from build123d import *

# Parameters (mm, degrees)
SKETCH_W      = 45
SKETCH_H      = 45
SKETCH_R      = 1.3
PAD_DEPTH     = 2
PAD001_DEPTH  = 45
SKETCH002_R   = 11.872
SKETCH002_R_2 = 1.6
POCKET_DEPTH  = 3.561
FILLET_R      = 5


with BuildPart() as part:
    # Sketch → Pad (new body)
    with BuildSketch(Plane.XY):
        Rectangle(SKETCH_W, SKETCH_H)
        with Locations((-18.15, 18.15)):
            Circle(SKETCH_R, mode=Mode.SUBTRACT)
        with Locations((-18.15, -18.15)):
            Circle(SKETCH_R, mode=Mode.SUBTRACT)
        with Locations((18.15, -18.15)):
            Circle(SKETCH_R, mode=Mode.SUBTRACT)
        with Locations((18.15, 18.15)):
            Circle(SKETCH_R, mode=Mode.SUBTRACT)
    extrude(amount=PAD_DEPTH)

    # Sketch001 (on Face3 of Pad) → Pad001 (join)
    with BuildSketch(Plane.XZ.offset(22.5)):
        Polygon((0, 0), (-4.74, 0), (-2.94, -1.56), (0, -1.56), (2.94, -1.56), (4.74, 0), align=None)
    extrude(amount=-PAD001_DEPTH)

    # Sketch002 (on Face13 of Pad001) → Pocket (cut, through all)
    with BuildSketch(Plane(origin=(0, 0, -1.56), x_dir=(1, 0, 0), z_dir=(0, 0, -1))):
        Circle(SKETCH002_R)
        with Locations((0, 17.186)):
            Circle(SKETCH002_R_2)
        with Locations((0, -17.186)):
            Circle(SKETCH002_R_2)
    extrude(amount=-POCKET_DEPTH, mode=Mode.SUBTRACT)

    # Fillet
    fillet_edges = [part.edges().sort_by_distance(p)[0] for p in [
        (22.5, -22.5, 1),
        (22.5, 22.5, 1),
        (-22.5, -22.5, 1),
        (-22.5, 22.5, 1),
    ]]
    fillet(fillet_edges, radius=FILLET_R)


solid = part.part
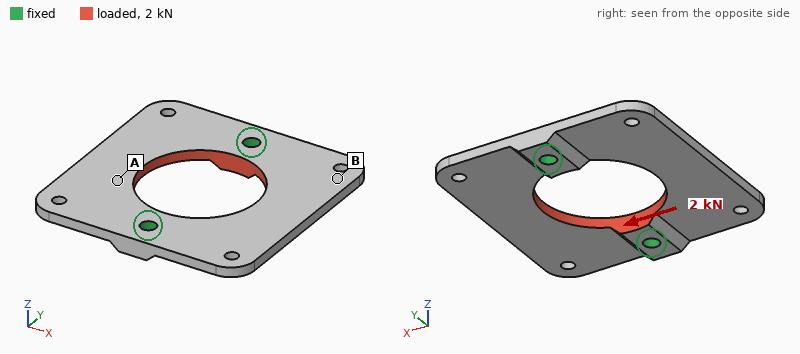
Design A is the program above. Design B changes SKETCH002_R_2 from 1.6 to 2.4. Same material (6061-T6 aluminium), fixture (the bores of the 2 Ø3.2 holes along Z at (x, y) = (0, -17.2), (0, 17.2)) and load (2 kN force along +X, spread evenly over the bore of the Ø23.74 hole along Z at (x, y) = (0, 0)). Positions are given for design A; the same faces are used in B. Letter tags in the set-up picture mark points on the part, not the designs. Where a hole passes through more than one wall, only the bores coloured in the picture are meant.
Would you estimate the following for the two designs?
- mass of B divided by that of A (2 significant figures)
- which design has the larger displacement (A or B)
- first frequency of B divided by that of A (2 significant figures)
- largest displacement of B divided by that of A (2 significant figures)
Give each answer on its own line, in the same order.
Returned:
0.98
A
1.0
0.79
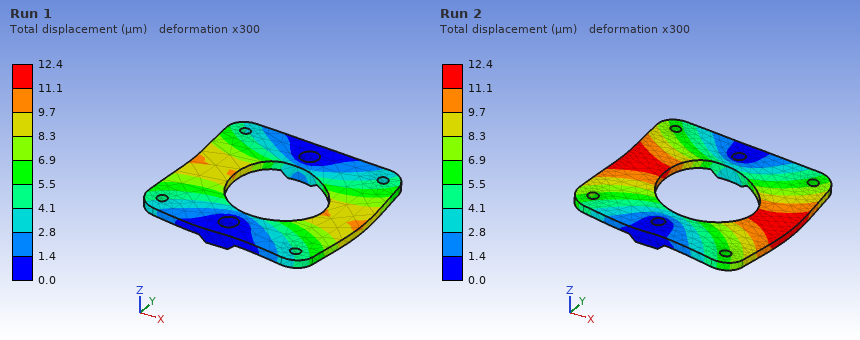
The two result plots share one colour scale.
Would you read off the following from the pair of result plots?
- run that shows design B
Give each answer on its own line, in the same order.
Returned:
Run 1
